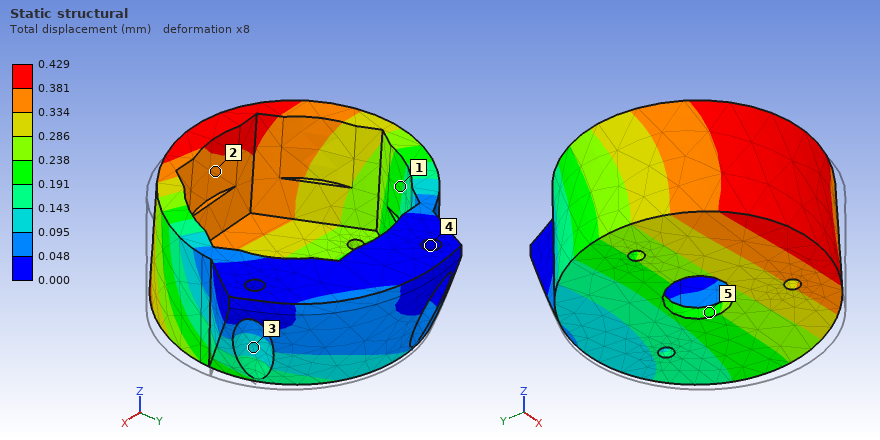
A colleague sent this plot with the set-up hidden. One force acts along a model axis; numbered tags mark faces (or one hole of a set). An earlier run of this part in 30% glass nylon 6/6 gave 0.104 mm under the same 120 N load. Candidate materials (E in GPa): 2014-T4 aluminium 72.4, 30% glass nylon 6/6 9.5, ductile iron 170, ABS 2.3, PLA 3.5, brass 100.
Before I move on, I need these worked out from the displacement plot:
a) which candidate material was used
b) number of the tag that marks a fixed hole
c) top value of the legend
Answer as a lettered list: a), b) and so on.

a) ABS
b) 4
c) 0.429 mm
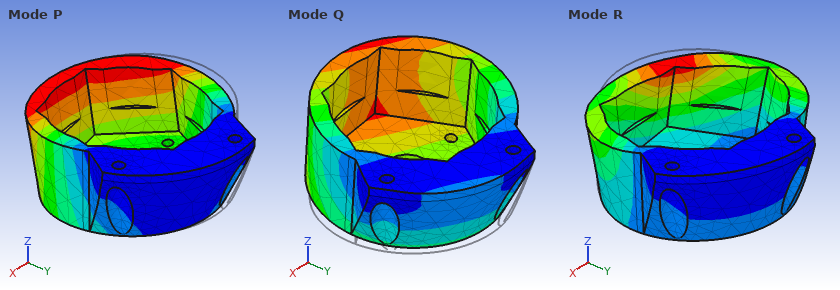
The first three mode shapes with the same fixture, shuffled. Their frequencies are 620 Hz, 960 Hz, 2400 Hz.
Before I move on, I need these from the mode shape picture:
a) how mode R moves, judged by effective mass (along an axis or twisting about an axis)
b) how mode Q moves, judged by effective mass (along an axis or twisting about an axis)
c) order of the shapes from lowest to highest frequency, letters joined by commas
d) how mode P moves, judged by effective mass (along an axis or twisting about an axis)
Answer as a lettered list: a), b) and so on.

a) along Y
b) along Z
c) Q, P, R
d) along X
